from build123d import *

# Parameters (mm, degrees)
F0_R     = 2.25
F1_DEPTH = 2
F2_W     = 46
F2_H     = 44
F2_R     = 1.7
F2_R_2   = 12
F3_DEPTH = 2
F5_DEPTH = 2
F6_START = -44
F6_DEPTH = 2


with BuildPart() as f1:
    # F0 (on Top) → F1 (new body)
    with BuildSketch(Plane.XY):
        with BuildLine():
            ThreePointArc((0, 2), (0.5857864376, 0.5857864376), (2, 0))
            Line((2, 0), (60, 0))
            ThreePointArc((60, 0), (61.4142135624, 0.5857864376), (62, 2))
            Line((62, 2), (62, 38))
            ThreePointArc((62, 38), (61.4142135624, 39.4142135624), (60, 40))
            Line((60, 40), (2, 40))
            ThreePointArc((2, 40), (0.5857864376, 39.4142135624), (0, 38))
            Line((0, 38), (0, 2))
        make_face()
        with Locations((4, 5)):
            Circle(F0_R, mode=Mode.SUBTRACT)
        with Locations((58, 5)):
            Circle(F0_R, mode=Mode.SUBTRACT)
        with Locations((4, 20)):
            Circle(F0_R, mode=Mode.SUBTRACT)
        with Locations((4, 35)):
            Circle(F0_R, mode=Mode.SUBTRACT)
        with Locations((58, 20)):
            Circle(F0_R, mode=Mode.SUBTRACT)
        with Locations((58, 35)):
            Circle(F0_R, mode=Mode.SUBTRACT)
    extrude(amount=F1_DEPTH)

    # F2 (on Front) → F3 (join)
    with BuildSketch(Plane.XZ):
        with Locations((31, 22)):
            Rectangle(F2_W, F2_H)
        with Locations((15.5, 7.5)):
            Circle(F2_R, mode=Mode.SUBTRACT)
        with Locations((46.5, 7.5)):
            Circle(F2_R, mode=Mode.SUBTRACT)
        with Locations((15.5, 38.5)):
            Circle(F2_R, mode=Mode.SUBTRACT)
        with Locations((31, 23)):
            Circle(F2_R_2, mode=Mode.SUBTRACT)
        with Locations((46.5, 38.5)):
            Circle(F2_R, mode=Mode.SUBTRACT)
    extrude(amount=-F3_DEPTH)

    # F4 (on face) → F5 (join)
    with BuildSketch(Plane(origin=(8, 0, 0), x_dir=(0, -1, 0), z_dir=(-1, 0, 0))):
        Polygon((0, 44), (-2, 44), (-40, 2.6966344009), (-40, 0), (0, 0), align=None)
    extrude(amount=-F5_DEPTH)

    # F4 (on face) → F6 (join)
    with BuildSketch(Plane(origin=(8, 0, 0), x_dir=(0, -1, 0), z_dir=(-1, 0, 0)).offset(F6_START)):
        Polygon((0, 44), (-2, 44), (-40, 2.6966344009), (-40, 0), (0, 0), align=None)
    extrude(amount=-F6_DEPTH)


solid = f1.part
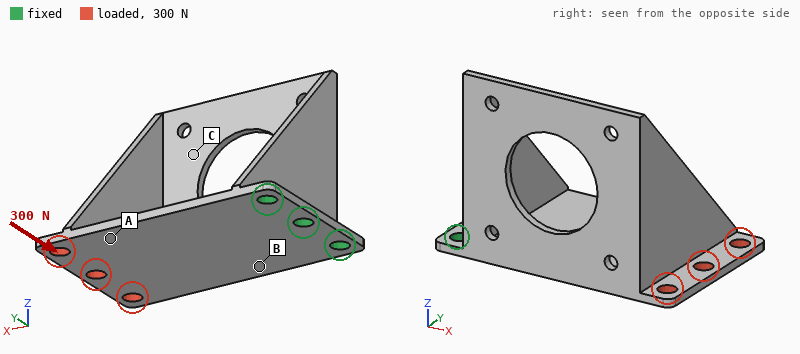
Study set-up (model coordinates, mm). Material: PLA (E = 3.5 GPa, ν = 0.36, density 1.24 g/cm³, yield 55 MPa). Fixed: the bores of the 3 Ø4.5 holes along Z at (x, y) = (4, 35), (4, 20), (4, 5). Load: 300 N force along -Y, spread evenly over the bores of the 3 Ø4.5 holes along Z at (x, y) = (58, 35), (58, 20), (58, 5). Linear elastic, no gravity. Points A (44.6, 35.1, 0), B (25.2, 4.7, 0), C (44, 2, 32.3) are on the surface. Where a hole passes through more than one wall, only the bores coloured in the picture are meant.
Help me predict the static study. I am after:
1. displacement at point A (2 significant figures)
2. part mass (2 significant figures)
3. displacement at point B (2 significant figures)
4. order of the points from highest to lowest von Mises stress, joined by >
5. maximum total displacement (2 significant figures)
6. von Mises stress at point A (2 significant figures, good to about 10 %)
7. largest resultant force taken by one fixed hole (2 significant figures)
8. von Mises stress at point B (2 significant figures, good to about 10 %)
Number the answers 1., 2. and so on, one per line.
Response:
1. 0.44 mm
2. 14 g
3. 0.19 mm
4. B > A > C
5. 0.74 mm
6. 6.0 MPa
7. 520 N
8. 11 MPa
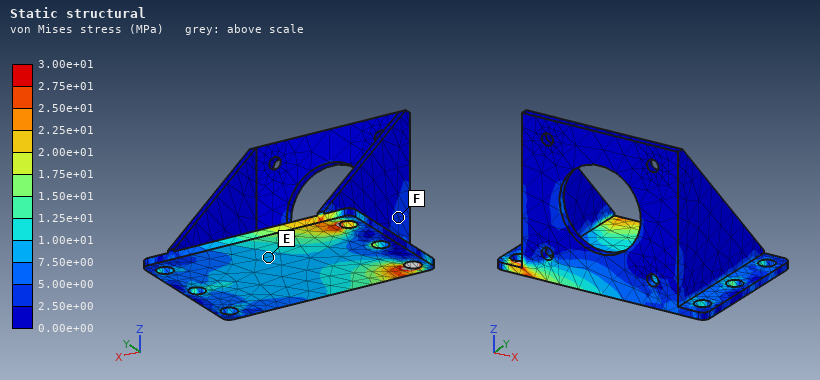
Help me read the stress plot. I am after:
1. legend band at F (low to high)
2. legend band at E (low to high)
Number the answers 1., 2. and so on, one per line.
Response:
1. 2.50e+00 to 5.00e+00 MPa
2. 7.50e+00 to 1.00e+01 MPa
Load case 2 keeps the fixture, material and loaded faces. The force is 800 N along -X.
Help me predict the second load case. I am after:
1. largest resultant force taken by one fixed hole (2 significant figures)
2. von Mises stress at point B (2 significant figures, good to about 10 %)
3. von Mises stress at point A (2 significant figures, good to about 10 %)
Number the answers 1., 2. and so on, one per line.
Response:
1. 270 N
2. 7.7 MPa
3. 11 MPa
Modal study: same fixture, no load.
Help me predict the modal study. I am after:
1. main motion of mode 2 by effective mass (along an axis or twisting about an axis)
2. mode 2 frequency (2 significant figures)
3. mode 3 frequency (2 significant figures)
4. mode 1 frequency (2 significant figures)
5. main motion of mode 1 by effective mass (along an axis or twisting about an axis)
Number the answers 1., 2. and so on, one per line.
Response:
1. along Y
2. 330 Hz
3. 1100 Hz
4. 150 Hz
5. along Z
